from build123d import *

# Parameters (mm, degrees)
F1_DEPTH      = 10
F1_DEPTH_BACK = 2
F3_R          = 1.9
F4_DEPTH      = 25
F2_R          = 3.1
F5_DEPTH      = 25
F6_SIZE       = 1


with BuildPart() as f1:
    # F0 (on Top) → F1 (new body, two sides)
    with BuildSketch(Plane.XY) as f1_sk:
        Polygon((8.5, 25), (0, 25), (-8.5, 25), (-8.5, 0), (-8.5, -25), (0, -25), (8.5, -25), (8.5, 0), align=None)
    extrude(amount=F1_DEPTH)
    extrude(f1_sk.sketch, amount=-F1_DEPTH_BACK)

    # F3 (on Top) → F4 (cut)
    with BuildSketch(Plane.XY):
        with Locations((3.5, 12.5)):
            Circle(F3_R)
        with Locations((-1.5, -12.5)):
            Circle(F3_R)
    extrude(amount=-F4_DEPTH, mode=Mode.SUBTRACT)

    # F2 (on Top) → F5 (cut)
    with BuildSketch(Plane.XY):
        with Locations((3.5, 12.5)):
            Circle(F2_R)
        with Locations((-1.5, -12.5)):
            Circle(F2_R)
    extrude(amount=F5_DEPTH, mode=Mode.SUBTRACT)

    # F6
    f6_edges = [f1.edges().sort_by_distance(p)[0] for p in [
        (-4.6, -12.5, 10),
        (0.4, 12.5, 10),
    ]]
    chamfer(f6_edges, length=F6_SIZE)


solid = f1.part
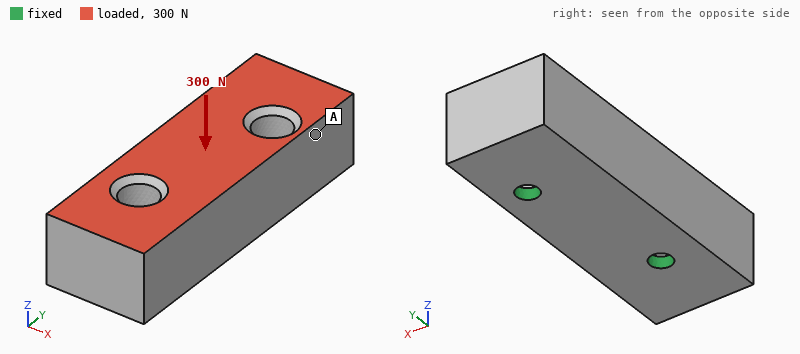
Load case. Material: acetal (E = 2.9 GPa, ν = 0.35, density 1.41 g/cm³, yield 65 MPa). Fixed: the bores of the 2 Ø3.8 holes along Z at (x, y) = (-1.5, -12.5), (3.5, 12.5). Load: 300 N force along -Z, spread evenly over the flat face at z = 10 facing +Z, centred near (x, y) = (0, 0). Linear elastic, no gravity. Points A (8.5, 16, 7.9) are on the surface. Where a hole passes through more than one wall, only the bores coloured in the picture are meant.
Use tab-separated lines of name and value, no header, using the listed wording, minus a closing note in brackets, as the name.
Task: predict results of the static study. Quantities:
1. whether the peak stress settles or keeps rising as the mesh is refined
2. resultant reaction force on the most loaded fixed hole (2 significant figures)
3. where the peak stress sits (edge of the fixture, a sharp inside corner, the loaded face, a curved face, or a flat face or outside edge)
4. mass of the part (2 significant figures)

whether the peak stress settles or keeps rising as the mesh is refined	keeps rising
resultant reaction force on the most loaded fixed hole	150 N
where the peak stress sits	edge of the fixture
mass of the part	13 g
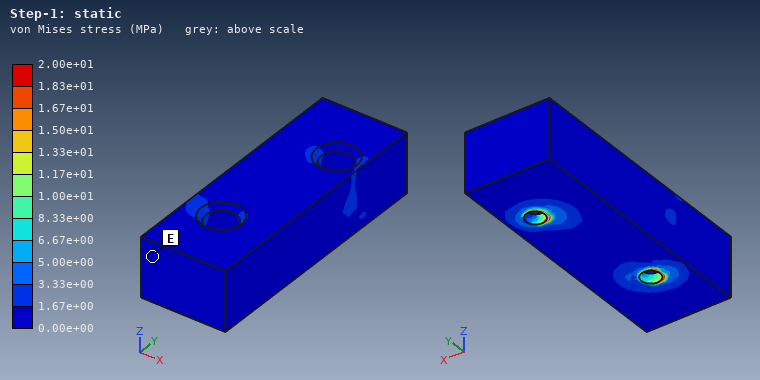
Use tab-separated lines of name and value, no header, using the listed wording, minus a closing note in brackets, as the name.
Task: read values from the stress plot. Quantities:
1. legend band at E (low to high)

legend band at E	0.00e+00 to 1.67e+00 MPa
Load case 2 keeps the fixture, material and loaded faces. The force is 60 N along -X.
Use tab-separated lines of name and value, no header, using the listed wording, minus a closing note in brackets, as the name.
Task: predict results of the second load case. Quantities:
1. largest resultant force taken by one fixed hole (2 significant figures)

largest resultant force taken by one fixed hole	30 N
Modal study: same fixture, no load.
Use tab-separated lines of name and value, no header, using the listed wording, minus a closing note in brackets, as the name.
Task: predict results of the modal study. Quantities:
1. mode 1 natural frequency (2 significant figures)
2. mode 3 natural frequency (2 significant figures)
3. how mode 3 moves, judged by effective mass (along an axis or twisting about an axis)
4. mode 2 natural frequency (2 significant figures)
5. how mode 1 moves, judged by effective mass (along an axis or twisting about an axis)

mode 1 natural frequency	1700 Hz
mode 3 natural frequency	4700 Hz
how mode 3 moves, judged by effective mass	along Y
mode 2 natural frequency	4300 Hz
how mode 1 moves, judged by effective mass	along X
